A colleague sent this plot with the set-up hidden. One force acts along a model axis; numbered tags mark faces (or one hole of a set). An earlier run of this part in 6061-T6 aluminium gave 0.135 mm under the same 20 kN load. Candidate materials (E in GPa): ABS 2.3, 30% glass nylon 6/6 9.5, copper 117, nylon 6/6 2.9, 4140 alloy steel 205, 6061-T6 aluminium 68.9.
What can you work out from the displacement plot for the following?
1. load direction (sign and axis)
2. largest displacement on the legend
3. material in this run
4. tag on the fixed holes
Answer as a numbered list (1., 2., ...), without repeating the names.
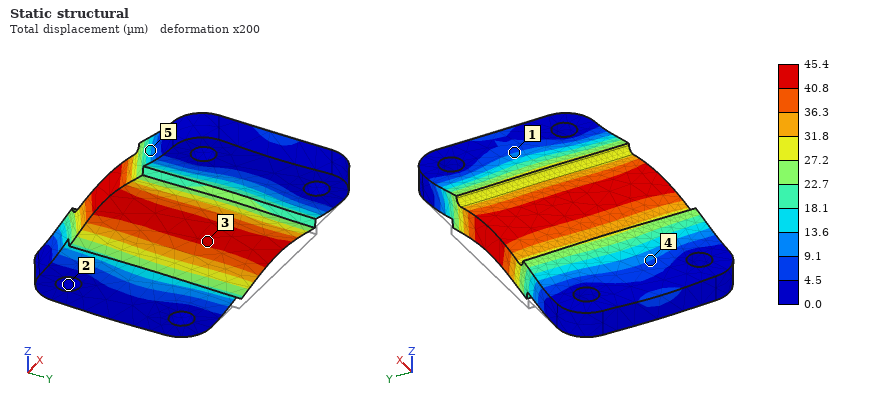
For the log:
1. +Z
2. 45.4 µm
3. 4140 alloy steel
4. 2
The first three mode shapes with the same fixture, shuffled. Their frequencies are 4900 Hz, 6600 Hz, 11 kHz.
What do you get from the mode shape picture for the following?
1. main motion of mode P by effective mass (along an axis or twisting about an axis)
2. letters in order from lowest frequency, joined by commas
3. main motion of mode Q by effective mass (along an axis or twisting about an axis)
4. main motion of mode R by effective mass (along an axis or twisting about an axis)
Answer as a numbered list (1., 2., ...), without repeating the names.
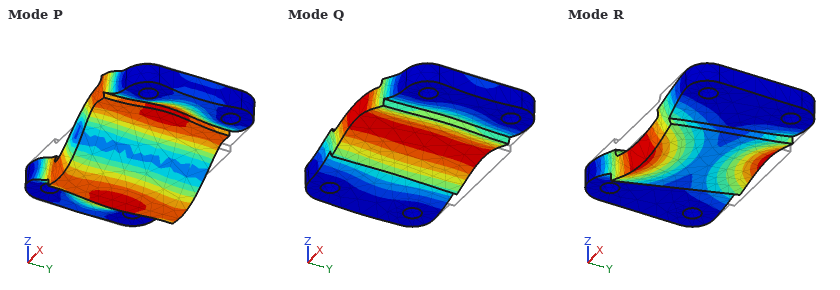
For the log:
1. twisting about Y
2. Q, R, P
3. along Z
4. twisting about X
